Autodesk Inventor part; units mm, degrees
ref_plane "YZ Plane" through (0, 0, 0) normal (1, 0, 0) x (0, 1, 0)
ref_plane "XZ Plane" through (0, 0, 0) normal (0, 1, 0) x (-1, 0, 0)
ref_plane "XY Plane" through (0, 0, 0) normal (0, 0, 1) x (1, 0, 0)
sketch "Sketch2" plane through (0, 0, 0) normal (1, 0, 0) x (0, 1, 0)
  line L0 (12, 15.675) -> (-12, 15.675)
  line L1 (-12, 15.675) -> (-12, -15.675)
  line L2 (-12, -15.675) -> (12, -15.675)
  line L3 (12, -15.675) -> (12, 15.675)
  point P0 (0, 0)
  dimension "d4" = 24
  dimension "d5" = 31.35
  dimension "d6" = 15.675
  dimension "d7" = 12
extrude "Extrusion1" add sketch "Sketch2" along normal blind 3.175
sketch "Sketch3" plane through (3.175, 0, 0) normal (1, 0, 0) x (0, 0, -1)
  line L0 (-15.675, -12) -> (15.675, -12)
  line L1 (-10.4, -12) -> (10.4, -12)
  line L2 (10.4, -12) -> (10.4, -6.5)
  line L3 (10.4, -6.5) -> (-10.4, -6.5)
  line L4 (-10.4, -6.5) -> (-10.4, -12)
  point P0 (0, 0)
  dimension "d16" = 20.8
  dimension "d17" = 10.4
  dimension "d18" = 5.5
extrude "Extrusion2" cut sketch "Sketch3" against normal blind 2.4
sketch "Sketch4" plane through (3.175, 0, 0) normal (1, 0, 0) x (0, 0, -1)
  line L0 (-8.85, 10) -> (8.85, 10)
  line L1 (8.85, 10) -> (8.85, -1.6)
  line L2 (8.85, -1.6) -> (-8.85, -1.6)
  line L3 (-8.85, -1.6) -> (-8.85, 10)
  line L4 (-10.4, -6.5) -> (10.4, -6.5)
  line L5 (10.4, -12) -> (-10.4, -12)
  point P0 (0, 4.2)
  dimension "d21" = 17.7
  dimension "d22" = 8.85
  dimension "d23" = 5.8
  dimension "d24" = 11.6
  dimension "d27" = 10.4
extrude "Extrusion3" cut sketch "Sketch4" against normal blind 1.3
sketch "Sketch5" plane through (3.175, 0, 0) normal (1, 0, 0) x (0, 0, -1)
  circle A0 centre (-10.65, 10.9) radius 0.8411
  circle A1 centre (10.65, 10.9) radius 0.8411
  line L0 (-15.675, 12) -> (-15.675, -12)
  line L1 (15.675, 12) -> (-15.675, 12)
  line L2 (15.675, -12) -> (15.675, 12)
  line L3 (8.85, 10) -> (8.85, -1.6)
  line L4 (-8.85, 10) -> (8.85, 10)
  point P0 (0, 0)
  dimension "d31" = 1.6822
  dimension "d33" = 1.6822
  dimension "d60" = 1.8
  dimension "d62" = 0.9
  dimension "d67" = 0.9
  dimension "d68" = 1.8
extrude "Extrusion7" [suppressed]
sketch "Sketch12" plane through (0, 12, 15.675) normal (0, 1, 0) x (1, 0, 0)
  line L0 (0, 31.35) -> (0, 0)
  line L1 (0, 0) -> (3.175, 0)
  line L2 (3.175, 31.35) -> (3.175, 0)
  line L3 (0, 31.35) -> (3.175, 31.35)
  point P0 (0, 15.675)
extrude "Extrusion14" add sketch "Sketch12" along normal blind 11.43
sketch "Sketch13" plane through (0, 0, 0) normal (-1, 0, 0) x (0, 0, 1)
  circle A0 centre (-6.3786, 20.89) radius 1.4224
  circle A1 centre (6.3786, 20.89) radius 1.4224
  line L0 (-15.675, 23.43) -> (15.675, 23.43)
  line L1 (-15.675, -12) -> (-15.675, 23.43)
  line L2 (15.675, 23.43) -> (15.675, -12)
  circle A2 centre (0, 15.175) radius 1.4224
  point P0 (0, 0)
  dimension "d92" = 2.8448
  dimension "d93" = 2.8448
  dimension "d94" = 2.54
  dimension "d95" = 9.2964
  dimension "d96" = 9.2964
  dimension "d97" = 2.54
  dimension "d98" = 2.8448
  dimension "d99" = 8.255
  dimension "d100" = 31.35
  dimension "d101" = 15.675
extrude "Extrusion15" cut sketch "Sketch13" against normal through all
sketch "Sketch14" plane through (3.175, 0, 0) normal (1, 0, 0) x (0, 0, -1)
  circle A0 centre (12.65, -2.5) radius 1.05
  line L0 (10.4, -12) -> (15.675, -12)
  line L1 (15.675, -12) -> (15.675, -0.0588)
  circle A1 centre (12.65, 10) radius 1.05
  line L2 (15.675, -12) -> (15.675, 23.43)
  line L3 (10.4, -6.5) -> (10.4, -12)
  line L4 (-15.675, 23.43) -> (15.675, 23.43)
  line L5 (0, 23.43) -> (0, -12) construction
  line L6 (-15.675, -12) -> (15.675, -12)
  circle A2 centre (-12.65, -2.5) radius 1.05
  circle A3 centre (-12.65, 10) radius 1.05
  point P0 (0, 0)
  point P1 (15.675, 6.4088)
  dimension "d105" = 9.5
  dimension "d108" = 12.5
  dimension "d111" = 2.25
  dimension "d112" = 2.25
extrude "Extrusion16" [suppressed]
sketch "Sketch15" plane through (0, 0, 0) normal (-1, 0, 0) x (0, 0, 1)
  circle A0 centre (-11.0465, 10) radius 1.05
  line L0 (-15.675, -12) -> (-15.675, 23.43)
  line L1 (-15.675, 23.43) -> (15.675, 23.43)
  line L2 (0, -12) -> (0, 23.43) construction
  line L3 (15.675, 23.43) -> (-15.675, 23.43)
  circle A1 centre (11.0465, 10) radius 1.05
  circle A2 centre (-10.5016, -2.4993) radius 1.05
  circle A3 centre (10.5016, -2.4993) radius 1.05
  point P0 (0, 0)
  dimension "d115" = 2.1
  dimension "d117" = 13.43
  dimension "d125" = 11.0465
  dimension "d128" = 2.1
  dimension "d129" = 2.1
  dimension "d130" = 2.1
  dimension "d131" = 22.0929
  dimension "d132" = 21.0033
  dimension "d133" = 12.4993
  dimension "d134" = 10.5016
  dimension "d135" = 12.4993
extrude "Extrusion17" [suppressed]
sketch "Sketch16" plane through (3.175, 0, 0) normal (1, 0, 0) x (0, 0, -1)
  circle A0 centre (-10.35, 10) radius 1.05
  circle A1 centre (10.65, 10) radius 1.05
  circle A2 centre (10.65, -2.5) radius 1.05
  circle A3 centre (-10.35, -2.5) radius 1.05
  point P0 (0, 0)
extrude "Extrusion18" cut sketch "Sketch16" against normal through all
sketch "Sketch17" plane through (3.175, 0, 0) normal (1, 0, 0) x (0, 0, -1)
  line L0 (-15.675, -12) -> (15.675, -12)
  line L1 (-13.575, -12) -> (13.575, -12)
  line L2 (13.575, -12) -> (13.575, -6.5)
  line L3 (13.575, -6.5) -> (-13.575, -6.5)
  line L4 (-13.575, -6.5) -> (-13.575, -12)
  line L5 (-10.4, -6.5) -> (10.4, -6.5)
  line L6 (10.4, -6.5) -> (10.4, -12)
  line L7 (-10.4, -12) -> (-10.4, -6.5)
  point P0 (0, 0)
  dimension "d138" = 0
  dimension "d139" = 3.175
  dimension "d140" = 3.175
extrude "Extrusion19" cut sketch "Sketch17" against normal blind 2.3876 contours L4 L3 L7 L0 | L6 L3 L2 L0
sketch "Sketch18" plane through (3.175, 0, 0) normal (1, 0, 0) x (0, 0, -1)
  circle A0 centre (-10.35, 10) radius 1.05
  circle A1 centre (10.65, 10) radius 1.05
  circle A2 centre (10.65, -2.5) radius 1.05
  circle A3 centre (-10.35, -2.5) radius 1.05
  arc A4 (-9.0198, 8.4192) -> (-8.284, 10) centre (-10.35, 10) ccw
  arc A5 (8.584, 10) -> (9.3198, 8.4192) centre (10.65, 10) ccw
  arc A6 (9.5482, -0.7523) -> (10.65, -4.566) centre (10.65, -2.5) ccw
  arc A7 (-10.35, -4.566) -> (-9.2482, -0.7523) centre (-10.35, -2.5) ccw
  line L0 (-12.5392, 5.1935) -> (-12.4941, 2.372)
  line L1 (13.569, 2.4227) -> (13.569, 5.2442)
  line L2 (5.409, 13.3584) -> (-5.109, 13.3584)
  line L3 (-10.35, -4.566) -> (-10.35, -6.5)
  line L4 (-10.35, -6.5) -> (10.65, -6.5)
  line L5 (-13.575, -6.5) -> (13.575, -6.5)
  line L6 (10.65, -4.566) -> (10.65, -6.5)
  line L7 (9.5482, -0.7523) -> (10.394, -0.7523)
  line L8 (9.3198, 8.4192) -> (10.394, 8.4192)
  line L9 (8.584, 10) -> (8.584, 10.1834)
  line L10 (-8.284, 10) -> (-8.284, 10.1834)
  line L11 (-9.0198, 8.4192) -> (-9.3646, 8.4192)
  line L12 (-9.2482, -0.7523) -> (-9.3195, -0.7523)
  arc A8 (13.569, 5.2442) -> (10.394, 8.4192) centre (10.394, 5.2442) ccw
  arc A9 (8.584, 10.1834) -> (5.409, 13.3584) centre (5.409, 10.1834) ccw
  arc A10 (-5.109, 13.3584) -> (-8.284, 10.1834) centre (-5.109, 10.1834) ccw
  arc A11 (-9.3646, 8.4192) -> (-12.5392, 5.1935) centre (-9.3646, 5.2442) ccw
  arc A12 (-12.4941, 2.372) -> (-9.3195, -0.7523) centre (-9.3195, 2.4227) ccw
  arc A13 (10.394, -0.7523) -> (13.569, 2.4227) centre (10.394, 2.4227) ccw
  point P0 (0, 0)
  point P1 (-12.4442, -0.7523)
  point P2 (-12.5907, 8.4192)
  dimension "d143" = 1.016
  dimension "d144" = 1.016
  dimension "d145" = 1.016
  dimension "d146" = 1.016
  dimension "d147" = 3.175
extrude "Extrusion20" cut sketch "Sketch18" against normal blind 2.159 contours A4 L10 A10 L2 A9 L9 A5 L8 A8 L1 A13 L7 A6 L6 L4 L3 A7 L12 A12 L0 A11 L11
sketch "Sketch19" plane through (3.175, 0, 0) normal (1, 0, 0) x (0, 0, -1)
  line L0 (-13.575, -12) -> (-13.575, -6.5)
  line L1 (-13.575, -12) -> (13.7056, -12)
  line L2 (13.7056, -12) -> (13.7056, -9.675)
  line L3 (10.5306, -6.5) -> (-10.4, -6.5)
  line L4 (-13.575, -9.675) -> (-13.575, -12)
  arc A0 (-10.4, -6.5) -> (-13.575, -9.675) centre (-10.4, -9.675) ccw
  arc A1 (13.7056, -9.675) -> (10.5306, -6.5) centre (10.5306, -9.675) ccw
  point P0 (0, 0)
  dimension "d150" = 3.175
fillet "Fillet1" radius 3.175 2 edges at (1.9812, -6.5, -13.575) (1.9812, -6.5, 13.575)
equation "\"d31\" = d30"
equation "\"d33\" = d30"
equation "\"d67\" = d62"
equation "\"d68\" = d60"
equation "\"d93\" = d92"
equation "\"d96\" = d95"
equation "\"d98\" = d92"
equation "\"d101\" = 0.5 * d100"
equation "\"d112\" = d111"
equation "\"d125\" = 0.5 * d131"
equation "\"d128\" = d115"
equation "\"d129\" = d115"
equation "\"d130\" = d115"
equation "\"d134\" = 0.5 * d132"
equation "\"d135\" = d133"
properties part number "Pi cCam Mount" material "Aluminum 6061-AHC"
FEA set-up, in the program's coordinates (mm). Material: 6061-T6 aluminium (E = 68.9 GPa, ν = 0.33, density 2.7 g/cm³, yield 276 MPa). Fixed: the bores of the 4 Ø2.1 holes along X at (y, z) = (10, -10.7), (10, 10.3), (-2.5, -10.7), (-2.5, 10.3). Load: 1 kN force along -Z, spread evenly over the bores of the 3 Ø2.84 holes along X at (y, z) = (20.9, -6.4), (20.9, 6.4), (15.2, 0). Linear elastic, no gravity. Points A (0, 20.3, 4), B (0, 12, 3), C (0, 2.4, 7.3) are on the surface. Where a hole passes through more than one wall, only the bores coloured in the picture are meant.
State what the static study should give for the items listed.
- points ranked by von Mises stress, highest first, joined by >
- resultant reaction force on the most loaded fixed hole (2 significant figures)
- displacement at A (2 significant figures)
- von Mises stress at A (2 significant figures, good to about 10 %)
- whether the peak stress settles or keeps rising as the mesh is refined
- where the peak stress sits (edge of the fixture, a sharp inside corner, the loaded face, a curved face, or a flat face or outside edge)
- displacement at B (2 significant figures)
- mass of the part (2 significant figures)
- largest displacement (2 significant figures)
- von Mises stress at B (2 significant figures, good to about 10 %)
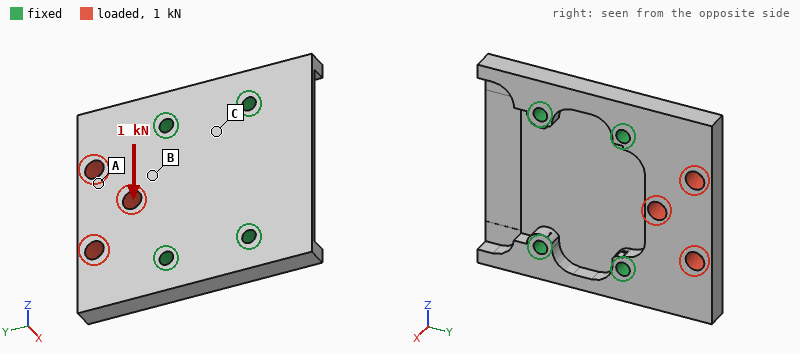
B > A > C
580 N
7.3 µm
15 MPa
keeps rising
edge of the fixture
3.4 µm
5.9 g
10 µm
32 MPa
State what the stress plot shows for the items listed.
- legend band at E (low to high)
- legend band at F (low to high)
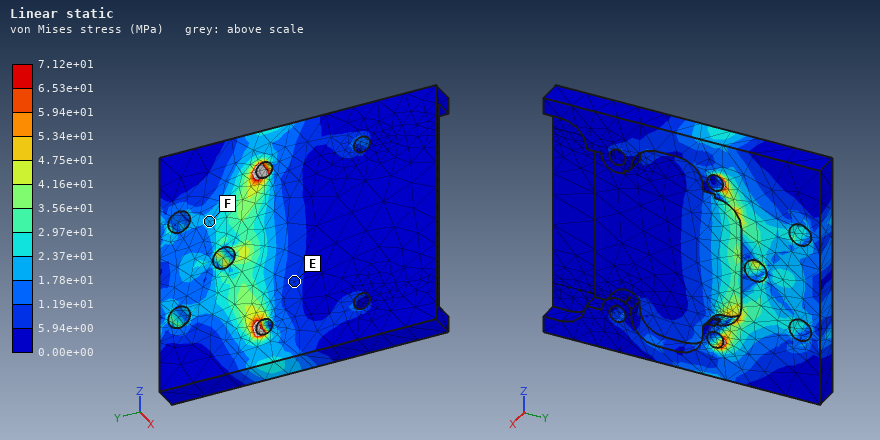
5.94e+00 to 1.19e+01 MPa
1.78e+01 to 2.37e+01 MPa
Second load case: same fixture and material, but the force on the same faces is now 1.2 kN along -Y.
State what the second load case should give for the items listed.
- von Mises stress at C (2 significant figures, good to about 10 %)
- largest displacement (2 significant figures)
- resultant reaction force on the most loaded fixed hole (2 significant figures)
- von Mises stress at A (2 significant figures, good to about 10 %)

13 MPa
11 µm
550 N
14 MPa
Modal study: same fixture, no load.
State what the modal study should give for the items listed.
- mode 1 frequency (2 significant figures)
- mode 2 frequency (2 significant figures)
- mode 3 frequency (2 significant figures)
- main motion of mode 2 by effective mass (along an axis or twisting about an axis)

10 kHz
11 kHz
17 kHz
along X
